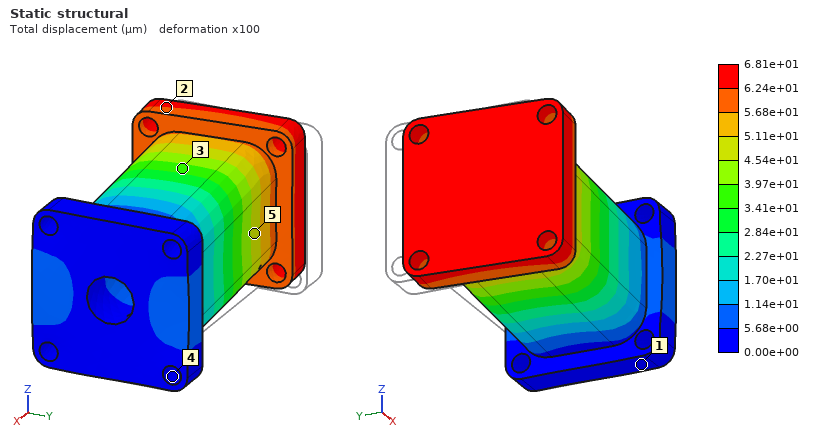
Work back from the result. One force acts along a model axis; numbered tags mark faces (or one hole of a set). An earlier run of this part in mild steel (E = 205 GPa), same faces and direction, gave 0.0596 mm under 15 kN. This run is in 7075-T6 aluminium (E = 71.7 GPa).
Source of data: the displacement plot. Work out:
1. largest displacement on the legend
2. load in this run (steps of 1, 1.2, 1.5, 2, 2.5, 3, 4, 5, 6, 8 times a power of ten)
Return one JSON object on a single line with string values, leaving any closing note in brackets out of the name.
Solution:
{"largest displacement on the legend": "6.81e+01 µm", "load in this run": "6 kN"}
